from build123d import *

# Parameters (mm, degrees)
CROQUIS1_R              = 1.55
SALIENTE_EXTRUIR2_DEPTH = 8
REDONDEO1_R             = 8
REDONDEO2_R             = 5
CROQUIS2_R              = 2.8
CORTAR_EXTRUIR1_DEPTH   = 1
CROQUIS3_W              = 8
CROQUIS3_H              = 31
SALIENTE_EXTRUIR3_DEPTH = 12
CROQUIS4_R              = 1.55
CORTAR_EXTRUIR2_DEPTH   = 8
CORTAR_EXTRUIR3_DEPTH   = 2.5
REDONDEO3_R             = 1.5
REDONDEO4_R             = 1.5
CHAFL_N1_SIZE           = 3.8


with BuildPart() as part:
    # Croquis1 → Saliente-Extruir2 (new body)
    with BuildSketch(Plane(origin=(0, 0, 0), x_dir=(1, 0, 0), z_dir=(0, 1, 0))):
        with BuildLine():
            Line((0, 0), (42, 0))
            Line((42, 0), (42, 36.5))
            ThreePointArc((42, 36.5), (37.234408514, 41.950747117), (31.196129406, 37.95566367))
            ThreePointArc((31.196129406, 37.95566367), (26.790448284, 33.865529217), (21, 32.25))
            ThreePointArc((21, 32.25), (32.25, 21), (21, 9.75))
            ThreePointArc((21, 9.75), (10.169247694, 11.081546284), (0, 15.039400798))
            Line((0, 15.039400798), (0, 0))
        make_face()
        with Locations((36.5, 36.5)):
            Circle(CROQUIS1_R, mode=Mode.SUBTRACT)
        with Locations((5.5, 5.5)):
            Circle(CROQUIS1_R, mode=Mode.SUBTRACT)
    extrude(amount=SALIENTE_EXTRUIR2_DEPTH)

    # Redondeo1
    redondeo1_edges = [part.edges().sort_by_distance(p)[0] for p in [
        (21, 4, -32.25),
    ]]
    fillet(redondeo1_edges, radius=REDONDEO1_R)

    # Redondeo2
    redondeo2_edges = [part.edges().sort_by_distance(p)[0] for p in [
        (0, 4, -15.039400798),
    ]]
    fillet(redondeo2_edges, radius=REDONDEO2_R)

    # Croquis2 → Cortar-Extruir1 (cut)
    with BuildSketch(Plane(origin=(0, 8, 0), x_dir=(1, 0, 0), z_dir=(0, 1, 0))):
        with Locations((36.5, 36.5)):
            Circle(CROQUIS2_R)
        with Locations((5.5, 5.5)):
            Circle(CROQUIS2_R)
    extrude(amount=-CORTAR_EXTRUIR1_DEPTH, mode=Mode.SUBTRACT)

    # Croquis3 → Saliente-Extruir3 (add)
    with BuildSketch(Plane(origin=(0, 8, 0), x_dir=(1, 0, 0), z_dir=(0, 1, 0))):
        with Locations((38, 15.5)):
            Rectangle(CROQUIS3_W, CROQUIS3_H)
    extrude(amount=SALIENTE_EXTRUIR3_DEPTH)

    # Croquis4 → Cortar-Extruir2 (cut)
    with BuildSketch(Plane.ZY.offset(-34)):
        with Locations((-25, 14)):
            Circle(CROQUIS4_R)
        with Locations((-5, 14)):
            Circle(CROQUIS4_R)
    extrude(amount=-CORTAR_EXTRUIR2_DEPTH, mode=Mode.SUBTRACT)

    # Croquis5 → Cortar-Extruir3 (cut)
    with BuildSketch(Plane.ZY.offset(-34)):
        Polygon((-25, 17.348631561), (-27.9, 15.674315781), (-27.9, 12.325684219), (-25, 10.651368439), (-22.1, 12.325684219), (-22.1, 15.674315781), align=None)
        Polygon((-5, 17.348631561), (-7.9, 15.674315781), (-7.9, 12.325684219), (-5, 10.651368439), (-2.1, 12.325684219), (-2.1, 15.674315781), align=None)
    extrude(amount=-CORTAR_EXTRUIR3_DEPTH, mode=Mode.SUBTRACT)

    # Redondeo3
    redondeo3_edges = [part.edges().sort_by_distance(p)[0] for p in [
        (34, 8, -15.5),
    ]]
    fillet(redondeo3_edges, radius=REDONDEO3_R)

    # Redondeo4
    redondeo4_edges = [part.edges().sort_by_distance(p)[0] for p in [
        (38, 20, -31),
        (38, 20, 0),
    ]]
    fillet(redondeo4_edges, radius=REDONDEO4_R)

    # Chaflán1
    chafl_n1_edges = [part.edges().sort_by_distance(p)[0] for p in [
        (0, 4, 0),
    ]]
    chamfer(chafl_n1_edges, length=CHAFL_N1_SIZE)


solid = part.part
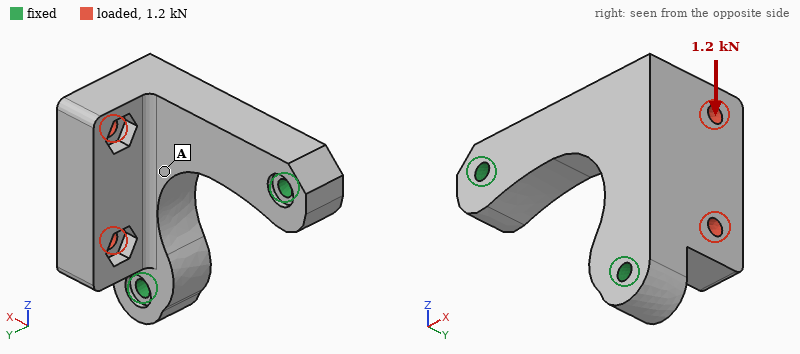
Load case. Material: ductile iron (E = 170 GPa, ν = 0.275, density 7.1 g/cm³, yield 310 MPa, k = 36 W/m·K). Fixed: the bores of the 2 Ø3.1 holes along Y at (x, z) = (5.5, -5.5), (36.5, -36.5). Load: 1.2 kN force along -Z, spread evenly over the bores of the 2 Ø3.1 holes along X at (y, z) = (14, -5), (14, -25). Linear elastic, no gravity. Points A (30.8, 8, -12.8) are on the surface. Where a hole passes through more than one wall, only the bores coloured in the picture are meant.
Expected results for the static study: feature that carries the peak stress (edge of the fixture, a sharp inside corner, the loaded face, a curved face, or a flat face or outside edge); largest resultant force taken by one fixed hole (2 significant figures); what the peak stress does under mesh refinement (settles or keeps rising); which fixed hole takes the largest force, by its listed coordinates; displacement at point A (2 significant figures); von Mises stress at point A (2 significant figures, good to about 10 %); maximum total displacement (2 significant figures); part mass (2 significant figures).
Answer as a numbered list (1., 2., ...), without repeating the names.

1. edge of the fixture
2. 1.2 kN
3. keeps rising
4. (36.5, -36.5)
5. 10 µm
6. 15 MPa
7. 27 µm
8. 64 g
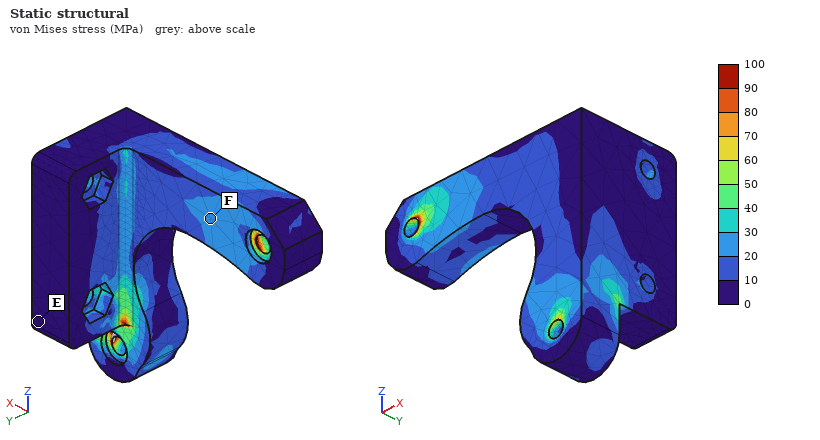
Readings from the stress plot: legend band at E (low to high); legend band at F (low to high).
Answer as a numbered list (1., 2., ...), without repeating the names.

1. 0 to 10 MPa
2. 20 to 30 MPa
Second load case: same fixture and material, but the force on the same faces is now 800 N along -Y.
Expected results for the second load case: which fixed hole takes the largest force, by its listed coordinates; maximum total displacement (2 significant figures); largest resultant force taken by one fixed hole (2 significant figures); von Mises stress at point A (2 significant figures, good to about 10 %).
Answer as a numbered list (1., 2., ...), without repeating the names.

1. (36.5, -36.5)
2. 37 µm
3. 560 N
4. 14 MPa
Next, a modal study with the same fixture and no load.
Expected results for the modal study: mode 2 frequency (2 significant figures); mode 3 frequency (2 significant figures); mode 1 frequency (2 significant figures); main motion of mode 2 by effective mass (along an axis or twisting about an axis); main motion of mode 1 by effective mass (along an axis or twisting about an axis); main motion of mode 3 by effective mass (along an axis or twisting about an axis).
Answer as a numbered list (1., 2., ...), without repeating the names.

1. 11 kHz
2. 20 kHz
3. 4700 Hz
4. along X
5. along Y
6. along Z
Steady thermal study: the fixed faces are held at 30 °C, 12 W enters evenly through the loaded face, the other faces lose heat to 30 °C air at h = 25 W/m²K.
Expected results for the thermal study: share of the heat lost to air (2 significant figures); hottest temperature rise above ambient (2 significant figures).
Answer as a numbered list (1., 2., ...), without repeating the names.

1. 17 %
2. 46 K
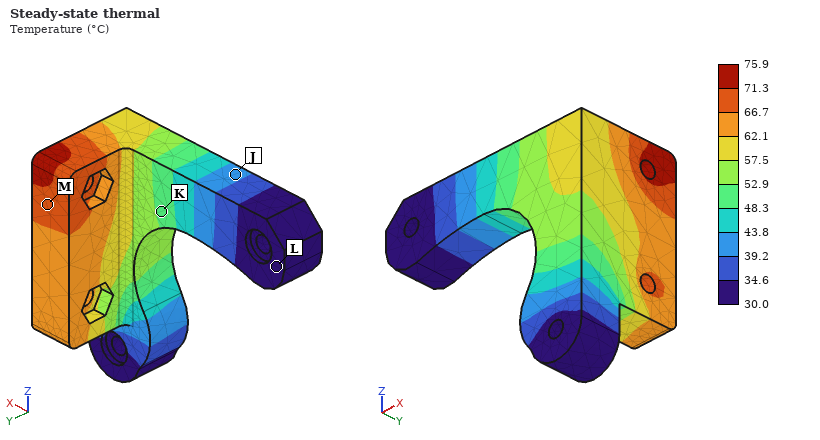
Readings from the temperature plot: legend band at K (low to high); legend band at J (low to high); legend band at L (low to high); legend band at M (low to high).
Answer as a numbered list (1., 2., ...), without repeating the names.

1. 48.3 to 52.9 °C
2. 39.2 to 43.8 °C
3. 30.0 to 34.6 °C
4. 66.7 to 71.3 °C
